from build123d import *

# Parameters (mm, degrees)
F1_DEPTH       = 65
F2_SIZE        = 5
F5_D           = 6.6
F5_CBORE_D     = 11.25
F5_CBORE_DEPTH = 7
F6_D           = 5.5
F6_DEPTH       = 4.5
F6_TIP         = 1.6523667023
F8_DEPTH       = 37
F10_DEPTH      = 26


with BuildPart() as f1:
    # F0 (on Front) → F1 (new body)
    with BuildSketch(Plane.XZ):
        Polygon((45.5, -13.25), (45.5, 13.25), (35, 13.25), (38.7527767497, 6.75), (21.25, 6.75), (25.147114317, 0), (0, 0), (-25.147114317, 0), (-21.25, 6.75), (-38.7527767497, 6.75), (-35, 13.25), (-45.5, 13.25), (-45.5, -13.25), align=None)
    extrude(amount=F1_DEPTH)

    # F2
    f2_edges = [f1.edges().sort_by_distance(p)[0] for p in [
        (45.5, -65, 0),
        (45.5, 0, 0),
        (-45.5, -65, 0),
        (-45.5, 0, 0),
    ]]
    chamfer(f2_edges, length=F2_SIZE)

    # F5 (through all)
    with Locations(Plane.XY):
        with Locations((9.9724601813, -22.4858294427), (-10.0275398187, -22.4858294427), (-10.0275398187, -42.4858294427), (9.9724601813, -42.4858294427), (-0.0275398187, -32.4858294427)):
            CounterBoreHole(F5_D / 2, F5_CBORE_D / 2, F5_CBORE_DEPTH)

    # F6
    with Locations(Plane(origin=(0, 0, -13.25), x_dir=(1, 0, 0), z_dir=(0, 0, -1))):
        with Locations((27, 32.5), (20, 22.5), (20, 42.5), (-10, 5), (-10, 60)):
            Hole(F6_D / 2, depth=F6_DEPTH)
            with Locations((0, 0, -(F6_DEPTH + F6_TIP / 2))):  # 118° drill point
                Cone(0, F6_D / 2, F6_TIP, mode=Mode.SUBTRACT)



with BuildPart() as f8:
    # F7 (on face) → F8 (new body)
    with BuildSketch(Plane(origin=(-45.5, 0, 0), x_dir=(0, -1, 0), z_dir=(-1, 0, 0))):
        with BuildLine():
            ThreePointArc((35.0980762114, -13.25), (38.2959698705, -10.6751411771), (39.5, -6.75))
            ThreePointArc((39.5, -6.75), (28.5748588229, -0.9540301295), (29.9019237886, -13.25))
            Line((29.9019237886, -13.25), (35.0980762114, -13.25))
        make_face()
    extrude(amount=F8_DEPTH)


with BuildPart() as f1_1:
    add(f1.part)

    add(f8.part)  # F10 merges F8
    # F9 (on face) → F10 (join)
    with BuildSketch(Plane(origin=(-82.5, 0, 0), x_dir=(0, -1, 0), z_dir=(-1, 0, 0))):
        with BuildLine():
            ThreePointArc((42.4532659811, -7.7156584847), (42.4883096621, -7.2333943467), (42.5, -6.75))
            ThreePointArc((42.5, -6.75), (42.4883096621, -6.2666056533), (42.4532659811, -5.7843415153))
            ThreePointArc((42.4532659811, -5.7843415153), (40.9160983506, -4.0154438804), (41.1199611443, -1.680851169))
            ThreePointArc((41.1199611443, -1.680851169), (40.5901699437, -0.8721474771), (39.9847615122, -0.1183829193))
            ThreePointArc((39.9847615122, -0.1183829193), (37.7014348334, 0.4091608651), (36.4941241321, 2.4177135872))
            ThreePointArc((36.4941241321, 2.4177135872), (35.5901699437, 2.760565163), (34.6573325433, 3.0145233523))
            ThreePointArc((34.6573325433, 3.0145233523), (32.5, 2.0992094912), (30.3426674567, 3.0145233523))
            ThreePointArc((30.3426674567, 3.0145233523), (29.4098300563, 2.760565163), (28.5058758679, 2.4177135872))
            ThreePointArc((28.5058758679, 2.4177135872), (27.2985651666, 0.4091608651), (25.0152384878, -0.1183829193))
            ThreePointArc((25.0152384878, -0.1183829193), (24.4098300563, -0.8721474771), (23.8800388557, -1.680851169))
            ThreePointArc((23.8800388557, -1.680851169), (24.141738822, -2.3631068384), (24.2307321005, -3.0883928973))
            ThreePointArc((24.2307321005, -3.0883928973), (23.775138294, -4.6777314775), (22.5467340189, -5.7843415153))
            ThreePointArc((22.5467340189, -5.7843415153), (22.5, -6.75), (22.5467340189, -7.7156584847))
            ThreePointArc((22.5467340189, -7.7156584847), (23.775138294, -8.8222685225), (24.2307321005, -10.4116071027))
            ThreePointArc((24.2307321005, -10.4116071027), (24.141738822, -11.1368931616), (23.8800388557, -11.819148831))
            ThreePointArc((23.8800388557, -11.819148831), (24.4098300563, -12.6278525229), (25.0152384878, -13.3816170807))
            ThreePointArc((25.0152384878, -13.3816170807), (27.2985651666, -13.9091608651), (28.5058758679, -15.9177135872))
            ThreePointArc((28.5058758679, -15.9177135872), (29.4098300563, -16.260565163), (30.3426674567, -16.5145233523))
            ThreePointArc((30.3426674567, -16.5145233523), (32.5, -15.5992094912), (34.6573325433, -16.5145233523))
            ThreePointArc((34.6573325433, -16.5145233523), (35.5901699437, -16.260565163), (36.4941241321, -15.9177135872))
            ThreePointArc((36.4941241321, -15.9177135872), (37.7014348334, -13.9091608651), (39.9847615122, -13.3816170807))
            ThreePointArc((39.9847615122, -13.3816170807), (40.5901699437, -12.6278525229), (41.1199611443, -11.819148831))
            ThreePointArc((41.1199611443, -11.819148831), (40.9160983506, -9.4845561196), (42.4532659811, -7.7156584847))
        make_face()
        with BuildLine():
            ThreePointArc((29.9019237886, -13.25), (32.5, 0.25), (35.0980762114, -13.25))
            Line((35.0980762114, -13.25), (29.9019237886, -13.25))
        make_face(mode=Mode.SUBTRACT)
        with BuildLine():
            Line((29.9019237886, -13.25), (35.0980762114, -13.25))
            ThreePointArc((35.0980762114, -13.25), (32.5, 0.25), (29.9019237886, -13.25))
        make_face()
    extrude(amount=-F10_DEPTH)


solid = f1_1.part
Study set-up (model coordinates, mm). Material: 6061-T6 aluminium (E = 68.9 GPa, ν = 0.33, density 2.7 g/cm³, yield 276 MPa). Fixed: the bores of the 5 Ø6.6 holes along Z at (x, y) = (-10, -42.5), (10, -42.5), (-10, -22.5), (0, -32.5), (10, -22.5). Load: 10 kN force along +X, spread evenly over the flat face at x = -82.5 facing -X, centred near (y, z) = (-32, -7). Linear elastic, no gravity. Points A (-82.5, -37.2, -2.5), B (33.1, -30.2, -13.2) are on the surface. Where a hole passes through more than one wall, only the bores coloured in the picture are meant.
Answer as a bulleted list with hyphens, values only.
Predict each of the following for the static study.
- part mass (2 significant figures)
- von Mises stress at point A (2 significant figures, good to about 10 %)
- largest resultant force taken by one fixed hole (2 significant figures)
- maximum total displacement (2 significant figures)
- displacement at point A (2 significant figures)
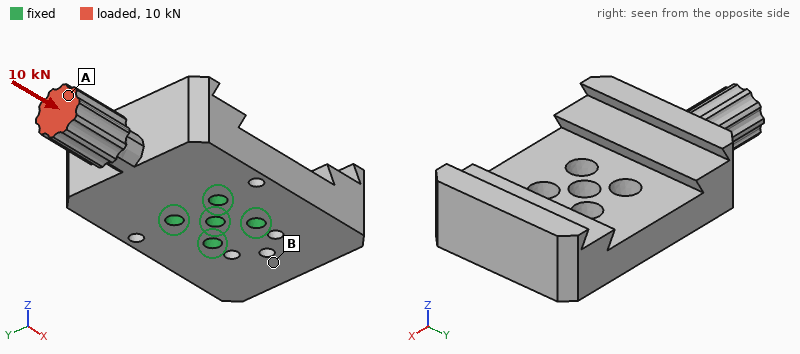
- 290 g
- 36 MPa
- 3.7 kN
- 43 µm
- 42 µm
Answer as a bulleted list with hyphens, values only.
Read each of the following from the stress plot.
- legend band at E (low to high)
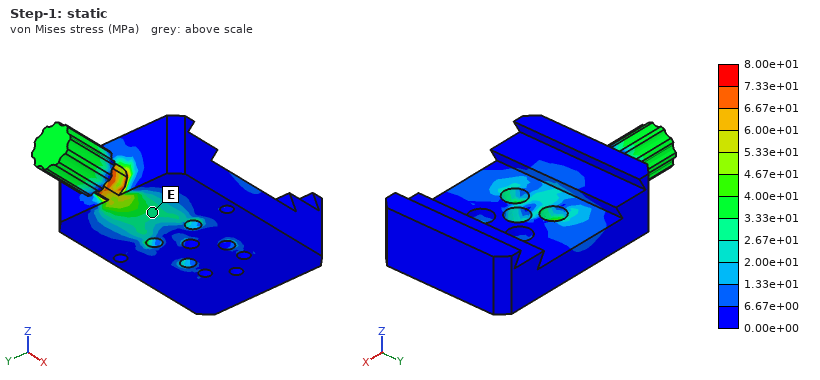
- 2.67e+01 to 3.33e+01 MPa
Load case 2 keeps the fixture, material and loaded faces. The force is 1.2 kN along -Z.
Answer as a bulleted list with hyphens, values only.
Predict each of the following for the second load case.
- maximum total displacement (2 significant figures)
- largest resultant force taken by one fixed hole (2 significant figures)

- 0.40 mm
- 2.5 kN
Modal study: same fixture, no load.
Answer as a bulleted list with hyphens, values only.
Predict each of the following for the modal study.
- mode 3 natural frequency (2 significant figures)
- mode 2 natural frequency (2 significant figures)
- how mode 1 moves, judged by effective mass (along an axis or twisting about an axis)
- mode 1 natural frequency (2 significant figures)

- 4000 Hz
- 3900 Hz
- along Z
- 2300 Hz
